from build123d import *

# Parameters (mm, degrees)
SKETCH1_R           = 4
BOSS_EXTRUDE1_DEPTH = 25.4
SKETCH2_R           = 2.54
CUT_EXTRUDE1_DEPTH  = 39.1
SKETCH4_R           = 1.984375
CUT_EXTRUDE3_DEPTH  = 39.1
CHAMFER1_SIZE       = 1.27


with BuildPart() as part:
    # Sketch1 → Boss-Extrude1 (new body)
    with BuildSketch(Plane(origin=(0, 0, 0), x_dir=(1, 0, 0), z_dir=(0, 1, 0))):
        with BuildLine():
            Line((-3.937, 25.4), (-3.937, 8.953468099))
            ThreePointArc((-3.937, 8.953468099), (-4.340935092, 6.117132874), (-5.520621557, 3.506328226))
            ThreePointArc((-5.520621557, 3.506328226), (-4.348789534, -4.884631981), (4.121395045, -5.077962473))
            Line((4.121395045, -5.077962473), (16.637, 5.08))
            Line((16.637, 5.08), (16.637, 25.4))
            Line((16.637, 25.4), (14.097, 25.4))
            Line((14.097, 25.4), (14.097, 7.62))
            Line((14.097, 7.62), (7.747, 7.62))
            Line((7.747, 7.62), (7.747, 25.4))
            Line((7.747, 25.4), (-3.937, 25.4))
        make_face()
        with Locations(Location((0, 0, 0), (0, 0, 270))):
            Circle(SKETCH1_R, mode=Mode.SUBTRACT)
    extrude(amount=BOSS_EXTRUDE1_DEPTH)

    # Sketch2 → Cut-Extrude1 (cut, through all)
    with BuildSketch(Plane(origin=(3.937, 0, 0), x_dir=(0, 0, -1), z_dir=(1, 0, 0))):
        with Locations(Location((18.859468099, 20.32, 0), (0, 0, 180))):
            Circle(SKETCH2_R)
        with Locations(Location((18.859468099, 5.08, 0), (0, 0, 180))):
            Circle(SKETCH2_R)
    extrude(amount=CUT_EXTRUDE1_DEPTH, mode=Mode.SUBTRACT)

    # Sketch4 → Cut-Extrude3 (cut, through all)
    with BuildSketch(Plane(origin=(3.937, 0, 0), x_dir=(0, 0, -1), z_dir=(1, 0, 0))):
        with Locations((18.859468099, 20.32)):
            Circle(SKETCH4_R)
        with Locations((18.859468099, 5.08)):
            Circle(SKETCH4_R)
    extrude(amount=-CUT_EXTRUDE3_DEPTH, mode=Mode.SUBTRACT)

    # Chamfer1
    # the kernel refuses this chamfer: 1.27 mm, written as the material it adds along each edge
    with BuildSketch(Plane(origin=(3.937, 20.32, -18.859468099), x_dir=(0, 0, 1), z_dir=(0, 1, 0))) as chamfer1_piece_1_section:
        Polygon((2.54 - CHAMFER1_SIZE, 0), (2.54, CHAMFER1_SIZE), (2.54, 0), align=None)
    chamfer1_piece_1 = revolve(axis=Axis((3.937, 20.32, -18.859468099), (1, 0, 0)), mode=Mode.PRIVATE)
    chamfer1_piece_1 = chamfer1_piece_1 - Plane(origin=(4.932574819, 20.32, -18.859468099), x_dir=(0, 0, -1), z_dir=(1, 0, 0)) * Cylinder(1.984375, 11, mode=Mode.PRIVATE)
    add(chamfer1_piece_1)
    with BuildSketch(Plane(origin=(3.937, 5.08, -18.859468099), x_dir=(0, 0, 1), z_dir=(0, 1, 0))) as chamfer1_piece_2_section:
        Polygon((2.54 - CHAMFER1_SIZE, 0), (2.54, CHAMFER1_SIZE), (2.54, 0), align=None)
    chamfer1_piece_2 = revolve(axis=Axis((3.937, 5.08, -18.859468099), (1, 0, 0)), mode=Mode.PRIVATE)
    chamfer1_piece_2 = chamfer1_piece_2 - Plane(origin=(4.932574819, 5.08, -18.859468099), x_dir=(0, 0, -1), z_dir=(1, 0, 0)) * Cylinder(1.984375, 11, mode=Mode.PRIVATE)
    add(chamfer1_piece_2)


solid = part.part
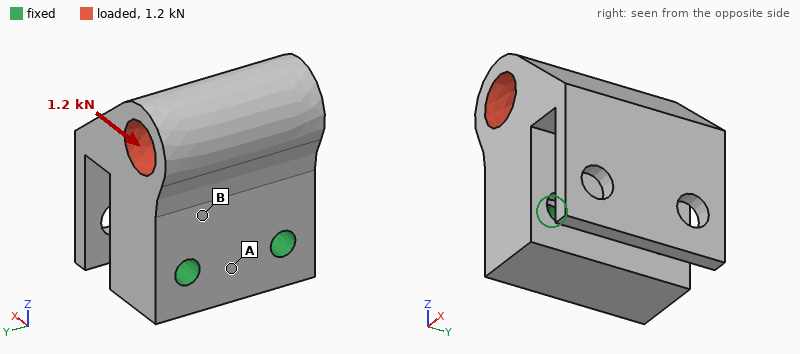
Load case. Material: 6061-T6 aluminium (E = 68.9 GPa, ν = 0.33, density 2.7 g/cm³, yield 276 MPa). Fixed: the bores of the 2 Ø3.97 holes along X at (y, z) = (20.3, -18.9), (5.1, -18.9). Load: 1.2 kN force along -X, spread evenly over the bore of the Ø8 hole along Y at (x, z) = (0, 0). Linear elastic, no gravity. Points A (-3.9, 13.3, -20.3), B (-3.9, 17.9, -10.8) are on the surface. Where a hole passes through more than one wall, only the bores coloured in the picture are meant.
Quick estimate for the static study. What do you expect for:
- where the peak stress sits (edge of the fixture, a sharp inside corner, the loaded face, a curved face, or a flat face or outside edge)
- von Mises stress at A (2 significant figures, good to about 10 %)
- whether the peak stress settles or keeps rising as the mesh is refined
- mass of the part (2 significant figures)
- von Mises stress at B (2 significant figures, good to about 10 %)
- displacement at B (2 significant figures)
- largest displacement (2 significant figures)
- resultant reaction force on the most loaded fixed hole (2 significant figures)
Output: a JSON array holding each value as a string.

["edge of the fixture", "11 MPa", "keeps rising", "28 g", "24 MPa", "8.3 µm", "32 µm", "600 N"]
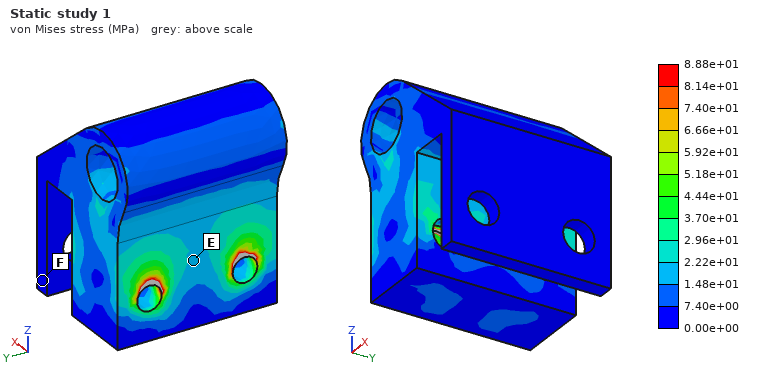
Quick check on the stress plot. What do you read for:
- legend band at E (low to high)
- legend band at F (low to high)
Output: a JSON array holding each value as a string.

["1.48e+01 to 2.22e+01 MPa", "0.00e+00 to 7.40e+00 MPa"]
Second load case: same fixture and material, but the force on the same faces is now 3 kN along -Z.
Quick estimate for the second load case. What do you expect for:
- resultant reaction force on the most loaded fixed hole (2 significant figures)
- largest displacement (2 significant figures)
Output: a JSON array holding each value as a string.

["1.5 kN", "12 µm"]
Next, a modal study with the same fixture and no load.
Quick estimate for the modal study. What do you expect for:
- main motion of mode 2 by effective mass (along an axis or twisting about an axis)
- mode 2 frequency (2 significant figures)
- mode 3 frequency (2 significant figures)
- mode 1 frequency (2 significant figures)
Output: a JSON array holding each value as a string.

["along X", "9700 Hz", "10 kHz", "5500 Hz"]
